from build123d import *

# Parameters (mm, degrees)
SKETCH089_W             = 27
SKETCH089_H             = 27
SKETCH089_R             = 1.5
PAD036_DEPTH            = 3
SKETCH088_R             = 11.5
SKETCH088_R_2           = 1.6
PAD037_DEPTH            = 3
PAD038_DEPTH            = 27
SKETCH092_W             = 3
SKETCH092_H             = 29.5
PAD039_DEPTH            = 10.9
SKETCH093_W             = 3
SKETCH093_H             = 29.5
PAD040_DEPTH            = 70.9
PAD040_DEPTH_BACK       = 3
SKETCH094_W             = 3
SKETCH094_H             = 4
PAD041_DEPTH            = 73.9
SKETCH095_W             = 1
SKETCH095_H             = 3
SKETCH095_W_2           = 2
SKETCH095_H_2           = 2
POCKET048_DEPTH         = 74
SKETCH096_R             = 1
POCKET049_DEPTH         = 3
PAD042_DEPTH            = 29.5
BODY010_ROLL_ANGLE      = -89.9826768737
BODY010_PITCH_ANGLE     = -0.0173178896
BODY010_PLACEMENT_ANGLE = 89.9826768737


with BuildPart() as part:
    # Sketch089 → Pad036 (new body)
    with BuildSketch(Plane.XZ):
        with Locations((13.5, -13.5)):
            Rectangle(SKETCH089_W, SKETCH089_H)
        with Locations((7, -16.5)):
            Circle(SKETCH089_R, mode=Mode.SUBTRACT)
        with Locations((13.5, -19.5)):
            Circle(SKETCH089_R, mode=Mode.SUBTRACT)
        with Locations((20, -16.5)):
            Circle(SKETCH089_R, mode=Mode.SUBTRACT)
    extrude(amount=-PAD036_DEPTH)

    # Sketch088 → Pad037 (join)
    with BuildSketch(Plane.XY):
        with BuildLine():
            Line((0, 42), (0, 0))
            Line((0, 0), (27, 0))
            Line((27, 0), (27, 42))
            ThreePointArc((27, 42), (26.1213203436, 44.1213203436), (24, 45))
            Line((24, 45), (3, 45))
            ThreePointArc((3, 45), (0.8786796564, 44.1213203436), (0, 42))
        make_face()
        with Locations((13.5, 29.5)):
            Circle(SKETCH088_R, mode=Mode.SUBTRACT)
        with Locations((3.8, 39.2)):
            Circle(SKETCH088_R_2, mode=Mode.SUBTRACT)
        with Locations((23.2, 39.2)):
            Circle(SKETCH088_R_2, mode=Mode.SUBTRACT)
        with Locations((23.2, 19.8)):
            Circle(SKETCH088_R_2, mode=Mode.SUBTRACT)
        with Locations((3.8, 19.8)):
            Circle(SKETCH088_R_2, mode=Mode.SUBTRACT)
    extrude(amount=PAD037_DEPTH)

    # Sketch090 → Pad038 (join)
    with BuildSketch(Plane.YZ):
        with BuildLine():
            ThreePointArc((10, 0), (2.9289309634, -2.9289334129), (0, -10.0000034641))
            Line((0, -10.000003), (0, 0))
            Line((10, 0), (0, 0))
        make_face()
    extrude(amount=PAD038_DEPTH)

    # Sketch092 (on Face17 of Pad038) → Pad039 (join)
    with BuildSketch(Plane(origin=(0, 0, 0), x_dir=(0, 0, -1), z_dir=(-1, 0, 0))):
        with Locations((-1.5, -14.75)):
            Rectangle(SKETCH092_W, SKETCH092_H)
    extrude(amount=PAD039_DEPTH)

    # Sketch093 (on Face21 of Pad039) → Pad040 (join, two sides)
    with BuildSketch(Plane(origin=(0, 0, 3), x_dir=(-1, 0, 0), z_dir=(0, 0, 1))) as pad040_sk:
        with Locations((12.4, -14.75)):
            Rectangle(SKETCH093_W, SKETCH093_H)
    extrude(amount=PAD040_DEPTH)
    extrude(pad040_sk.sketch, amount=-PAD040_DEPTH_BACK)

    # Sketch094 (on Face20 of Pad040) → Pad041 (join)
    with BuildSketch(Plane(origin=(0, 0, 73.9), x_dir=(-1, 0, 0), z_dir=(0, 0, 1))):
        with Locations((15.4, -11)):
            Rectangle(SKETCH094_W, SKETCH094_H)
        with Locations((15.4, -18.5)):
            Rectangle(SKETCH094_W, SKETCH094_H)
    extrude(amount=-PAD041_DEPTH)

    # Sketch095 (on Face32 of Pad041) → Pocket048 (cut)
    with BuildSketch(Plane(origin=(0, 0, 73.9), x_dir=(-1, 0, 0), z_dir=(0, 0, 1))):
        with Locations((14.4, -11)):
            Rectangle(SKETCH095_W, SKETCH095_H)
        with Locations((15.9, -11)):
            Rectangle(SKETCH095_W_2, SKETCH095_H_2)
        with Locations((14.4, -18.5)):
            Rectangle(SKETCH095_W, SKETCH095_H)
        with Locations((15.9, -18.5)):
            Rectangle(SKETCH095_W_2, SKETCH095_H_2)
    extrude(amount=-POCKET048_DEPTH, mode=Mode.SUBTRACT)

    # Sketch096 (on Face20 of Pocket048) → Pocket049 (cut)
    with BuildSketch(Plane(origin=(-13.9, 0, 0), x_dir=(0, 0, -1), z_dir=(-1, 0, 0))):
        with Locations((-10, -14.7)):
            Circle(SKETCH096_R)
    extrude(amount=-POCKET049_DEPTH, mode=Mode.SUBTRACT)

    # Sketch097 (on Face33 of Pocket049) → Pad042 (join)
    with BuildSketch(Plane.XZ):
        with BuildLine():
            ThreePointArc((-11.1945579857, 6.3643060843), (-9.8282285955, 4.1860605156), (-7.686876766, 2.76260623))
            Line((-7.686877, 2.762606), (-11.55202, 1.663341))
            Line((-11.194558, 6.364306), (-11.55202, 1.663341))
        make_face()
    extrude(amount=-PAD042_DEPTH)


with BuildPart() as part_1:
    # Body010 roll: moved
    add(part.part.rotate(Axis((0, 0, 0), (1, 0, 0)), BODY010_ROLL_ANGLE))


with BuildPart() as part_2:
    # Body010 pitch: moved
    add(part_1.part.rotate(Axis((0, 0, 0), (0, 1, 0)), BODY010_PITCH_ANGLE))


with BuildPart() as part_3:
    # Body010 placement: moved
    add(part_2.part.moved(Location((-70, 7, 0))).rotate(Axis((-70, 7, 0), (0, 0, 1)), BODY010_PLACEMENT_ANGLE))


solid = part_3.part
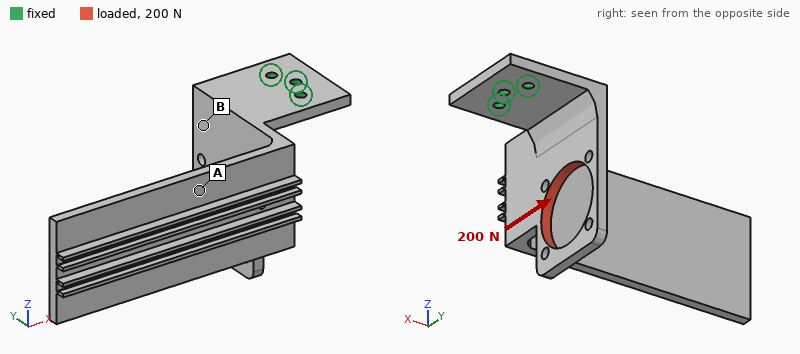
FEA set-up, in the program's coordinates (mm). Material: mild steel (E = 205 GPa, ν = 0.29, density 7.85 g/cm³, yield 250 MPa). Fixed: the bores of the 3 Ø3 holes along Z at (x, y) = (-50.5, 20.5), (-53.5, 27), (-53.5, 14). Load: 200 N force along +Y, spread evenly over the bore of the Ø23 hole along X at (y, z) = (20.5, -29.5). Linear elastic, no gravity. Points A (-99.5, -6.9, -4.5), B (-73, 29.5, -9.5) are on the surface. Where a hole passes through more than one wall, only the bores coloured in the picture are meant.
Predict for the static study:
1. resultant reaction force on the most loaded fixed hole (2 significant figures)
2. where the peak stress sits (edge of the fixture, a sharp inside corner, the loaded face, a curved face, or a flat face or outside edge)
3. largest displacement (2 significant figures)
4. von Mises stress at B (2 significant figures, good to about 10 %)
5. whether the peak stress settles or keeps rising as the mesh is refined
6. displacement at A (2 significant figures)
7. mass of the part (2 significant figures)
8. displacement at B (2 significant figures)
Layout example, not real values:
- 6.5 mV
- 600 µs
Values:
- 420 N
- edge of the fixture
- 0.11 mm
- 18 MPa
- keeps rising
- 0.079 mm
- 100 g
- 0.027 mm
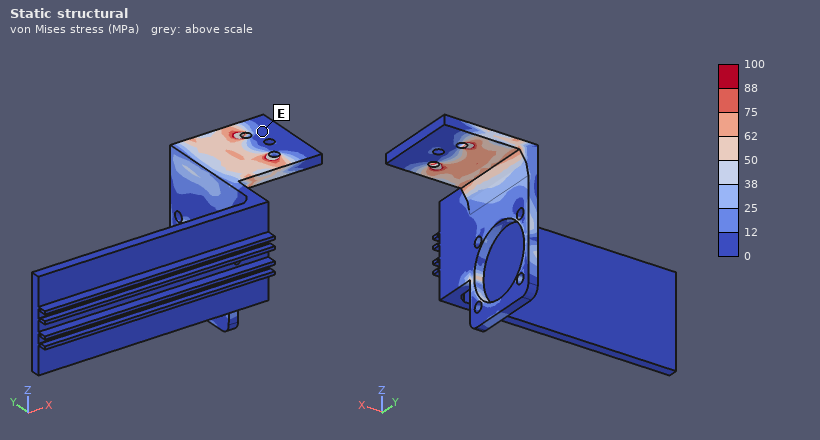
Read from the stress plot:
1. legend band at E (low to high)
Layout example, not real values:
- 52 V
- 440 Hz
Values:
- 0 to 12 MPa
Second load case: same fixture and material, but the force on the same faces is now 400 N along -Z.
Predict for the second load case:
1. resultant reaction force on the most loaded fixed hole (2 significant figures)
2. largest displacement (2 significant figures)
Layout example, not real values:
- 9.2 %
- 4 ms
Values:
- 280 N
- 0.43 mm
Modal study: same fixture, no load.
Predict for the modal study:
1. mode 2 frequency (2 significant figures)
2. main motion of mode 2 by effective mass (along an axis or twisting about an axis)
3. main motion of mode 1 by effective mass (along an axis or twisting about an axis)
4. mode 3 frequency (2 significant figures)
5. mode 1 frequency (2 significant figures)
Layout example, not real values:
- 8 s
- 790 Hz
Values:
- 370 Hz
- along Y
- along Z
- 1400 Hz
- 270 Hz
